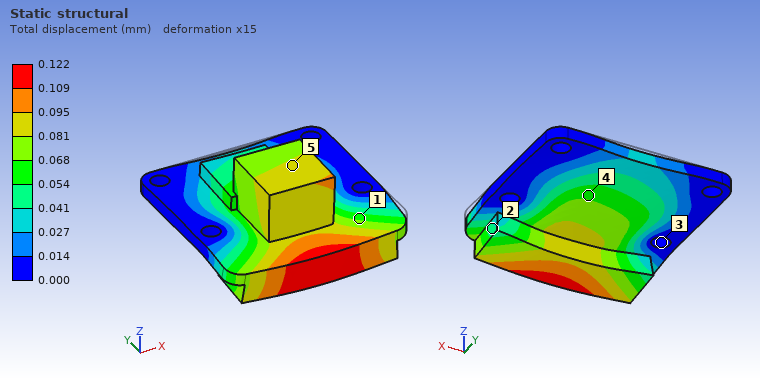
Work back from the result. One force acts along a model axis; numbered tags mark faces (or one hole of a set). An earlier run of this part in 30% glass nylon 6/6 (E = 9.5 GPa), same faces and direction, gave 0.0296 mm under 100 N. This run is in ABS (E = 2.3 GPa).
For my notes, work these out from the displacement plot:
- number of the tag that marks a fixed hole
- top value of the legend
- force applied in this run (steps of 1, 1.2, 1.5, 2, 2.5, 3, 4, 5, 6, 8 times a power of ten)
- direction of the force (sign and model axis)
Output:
3
0.122 mm
100 N
-Z
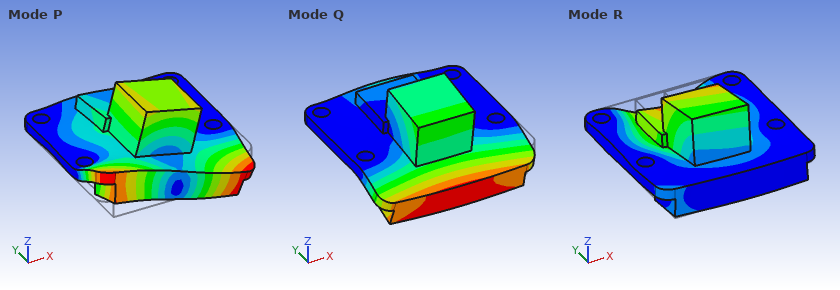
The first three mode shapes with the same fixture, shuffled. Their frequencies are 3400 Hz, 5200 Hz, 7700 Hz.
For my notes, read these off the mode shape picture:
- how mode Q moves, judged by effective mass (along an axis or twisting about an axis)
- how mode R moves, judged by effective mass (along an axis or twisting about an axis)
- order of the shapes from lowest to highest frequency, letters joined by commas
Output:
along Z
along Z
Q, R, P
